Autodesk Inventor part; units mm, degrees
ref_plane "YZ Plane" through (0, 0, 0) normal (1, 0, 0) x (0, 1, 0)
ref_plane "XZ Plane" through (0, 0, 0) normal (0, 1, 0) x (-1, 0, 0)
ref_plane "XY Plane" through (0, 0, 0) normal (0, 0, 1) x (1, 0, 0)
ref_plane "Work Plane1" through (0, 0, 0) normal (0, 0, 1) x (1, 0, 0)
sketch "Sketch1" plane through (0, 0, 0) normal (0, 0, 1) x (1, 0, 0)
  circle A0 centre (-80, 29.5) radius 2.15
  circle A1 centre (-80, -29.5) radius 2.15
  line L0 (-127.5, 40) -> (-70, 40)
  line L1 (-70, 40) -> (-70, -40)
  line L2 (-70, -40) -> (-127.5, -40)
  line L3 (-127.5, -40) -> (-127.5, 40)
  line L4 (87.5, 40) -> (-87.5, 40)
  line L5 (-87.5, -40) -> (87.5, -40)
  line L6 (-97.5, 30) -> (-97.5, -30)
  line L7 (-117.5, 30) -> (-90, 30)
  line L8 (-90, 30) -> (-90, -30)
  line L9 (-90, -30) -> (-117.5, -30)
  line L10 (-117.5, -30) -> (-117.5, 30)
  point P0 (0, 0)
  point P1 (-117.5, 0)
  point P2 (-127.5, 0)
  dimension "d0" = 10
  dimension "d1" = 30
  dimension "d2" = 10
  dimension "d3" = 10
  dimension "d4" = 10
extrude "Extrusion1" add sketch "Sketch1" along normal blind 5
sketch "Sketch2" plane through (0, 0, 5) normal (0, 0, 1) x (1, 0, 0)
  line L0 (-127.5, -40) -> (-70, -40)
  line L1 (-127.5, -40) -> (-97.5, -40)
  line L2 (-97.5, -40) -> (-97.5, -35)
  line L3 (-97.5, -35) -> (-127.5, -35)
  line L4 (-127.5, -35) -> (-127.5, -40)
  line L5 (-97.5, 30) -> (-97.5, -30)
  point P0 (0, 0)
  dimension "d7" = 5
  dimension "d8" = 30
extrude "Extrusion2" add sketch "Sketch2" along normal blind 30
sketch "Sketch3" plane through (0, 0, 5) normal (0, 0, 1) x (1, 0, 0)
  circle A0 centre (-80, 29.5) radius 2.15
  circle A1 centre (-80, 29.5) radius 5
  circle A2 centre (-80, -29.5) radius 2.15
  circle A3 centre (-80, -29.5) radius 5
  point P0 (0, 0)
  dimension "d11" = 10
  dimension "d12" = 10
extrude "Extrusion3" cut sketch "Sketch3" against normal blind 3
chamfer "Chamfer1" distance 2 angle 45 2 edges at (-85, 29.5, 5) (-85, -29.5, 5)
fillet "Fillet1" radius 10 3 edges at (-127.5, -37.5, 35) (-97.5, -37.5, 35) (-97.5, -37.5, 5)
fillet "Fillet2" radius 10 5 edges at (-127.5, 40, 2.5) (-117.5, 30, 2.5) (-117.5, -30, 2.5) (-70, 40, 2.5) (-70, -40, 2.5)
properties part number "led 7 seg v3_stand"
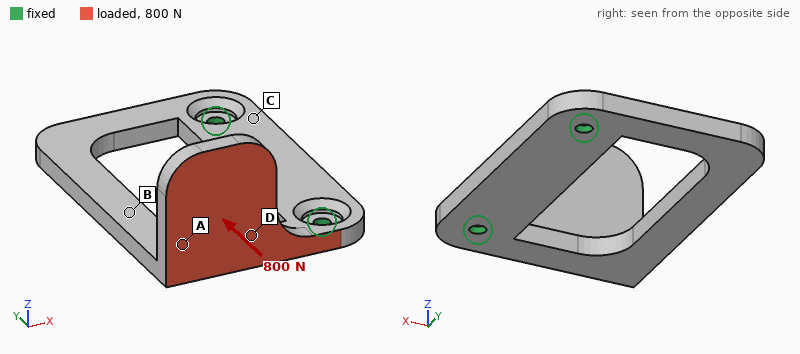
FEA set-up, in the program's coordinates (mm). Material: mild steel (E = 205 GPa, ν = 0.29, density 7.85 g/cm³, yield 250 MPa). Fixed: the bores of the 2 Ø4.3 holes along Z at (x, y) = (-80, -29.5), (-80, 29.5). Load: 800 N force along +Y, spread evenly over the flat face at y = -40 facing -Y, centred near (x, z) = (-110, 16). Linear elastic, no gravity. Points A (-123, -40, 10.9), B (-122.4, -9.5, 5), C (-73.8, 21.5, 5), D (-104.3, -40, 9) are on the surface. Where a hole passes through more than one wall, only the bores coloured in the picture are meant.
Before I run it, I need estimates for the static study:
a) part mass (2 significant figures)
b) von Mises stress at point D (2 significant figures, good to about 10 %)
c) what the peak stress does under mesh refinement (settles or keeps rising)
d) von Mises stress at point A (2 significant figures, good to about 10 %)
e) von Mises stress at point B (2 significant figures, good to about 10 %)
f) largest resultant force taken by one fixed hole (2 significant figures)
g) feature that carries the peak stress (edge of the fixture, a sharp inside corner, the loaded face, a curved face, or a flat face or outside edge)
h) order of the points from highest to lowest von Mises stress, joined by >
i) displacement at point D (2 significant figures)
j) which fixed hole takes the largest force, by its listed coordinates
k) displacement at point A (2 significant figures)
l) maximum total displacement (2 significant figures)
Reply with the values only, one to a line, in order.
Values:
140 g
58 MPa
keeps rising
38 MPa
77 MPa
850 N
edge of the fixture
B > D > A > C
0.092 mm
(-80, 29.5)
0.14 mm
0.27 mm
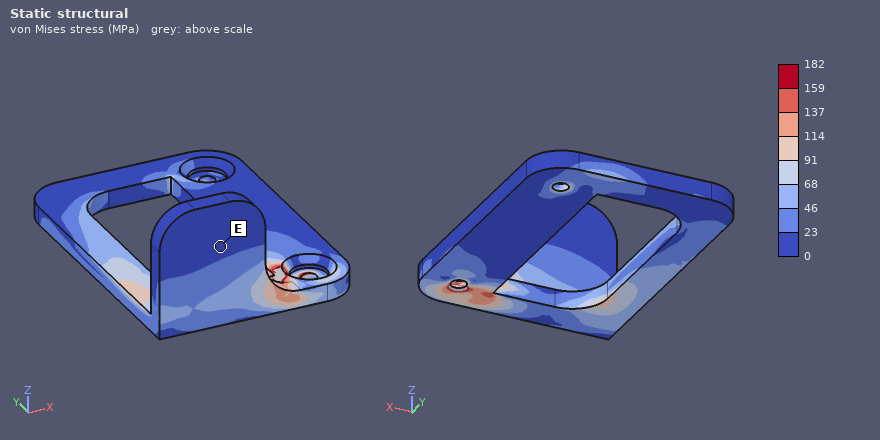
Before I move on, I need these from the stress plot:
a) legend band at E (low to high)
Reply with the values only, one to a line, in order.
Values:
0 to 23 MPa
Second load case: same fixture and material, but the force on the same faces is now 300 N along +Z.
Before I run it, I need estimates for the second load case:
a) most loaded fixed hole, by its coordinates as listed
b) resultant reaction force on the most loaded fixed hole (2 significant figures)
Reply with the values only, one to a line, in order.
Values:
(-80, -29.5)
380 N
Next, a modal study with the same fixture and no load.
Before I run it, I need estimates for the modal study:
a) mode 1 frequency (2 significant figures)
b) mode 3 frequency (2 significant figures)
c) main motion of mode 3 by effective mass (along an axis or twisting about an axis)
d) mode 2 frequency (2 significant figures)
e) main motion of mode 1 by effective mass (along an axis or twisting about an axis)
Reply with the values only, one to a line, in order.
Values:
660 Hz
2100 Hz
along Y
1300 Hz
along Z
